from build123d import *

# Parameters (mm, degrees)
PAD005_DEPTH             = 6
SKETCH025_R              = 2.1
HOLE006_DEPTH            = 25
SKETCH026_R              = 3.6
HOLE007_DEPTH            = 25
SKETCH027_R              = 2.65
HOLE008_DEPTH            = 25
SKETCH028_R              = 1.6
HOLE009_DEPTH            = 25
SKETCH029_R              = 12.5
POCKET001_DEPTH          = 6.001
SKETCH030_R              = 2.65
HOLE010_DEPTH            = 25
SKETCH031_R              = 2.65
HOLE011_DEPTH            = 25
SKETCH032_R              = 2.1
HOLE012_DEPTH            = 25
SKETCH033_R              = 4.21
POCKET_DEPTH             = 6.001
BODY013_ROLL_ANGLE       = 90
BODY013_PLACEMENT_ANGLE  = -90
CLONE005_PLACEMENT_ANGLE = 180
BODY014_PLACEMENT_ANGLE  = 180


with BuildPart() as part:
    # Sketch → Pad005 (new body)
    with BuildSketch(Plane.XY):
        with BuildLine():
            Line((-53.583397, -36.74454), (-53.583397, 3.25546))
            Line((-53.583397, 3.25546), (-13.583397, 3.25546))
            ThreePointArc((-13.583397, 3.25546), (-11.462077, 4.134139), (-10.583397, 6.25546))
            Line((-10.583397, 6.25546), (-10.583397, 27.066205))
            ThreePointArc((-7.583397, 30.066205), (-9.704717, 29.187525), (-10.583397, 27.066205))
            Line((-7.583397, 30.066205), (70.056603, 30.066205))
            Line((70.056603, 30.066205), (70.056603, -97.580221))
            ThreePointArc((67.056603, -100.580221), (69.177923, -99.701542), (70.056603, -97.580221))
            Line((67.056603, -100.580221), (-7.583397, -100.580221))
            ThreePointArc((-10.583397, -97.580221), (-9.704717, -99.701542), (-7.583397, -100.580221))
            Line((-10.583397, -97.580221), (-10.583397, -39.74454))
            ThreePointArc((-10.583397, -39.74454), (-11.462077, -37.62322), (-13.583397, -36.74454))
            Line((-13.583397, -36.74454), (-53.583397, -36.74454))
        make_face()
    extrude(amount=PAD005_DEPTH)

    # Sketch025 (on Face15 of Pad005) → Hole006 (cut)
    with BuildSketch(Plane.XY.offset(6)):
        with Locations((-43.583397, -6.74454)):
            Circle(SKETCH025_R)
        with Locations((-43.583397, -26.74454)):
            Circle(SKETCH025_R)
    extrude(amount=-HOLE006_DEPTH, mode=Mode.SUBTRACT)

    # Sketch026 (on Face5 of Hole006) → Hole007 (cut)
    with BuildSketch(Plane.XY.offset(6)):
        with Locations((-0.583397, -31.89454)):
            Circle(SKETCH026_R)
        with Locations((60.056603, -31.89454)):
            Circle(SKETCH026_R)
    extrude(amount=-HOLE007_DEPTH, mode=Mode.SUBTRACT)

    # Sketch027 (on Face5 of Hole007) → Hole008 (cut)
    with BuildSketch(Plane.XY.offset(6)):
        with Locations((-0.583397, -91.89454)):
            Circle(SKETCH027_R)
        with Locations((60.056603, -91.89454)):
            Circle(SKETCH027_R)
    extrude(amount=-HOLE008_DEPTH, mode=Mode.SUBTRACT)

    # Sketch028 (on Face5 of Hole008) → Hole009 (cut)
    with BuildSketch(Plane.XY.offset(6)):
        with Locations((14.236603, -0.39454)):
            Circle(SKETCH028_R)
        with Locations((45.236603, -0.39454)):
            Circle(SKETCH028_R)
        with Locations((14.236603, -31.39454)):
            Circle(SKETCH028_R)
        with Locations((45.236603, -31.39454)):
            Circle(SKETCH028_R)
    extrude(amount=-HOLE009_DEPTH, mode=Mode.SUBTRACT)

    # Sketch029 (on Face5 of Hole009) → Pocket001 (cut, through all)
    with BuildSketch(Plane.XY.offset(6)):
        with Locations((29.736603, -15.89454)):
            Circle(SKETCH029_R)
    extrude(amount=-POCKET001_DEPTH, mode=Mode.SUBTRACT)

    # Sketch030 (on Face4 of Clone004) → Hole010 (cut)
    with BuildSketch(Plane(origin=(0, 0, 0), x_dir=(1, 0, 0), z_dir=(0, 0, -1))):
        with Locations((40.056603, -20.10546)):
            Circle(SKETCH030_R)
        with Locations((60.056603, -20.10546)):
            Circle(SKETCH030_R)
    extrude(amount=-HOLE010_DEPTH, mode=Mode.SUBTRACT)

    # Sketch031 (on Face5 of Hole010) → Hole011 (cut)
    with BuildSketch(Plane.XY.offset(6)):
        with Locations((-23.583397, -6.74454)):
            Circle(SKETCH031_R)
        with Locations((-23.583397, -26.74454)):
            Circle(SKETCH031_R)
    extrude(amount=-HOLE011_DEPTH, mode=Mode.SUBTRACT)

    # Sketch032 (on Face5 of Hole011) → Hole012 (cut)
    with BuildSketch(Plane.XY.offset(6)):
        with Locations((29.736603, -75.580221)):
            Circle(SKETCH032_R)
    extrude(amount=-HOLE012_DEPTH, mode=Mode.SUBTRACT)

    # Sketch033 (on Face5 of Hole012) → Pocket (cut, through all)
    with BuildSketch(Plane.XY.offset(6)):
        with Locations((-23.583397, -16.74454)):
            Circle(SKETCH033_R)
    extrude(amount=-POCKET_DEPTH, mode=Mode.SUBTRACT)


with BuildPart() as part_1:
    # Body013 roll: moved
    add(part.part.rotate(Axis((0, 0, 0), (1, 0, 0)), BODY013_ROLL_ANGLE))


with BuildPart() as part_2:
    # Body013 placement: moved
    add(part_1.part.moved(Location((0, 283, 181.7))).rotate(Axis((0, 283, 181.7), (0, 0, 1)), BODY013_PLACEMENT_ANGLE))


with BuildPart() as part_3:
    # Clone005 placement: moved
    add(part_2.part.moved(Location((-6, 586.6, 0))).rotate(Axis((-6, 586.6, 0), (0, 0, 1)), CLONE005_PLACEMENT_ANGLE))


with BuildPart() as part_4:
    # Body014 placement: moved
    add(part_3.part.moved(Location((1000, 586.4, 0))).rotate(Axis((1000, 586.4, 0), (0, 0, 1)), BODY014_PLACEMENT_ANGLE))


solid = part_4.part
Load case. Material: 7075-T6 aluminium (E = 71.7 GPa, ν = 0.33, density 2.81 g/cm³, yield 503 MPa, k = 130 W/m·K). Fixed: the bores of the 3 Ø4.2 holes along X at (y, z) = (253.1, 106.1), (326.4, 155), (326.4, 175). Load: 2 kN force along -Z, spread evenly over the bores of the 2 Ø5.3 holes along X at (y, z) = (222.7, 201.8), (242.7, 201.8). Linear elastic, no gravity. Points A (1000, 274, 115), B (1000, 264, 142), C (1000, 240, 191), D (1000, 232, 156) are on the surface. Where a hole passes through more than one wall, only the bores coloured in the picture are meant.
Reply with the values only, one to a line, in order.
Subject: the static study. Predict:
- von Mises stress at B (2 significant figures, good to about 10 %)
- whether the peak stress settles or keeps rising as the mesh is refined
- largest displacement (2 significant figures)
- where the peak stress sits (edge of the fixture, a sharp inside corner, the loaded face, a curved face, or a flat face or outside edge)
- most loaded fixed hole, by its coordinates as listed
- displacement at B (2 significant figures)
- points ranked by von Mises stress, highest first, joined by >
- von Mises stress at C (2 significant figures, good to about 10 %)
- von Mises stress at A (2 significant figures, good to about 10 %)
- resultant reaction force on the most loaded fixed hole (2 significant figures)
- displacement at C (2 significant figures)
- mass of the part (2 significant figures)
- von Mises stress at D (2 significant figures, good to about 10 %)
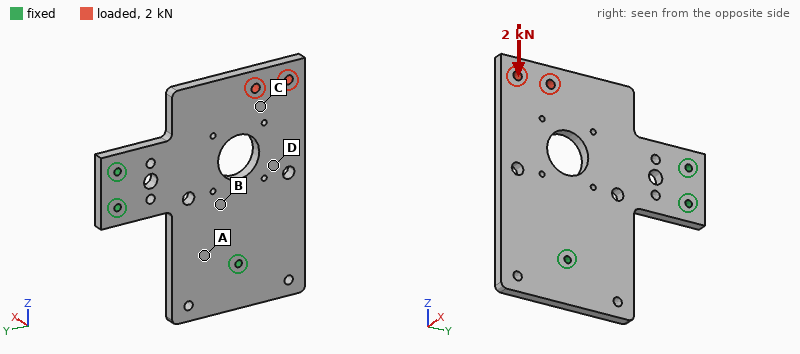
4.2 MPa
keeps rising
22 µm
edge of the fixture
(253.1, 106.1)
3.5 µm
D > C > B > A
8.0 MPa
2.2 MPa
2.1 kN
17 µm
190 g
11 MPa
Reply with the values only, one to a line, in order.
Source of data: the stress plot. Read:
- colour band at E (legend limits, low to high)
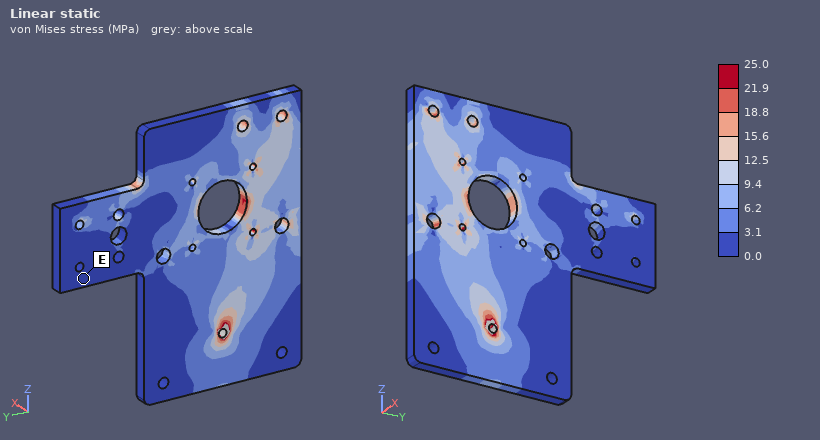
0.0 to 3.1 MPa
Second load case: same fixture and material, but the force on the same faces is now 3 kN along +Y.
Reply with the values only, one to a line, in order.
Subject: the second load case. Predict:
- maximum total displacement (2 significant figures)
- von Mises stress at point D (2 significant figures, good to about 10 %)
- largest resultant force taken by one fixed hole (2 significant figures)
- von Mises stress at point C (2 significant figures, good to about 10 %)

49 µm
8.5 MPa
1.9 kN
16 MPa
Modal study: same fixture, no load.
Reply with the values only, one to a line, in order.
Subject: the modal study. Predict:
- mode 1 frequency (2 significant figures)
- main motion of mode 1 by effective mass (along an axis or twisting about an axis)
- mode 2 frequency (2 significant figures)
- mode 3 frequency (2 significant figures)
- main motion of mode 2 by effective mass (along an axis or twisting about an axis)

570 Hz
along X
1800 Hz
2500 Hz
twisting about Z
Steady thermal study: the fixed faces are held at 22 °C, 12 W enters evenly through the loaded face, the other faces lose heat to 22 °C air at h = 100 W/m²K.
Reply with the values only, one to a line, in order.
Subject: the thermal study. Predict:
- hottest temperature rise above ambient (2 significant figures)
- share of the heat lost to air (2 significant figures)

14 K
72 %
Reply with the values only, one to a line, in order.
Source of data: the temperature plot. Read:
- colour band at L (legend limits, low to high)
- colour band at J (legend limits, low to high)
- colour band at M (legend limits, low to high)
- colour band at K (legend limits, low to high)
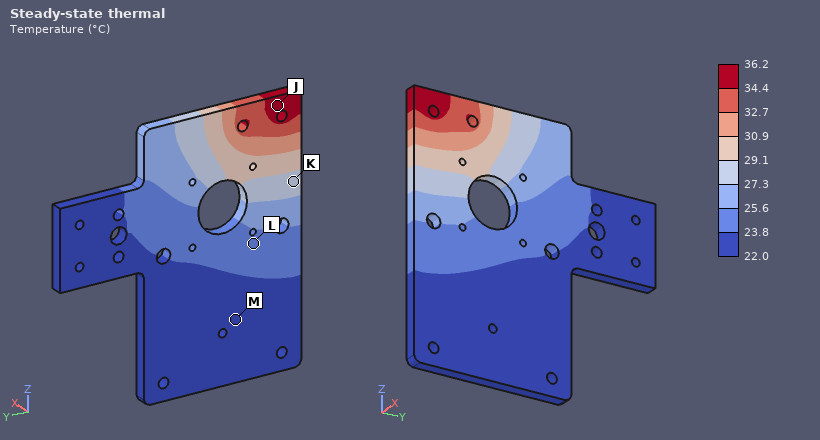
23.8 to 25.6 °C
34.4 to 36.2 °C
22.0 to 23.8 °C
27.3 to 29.1 °C
